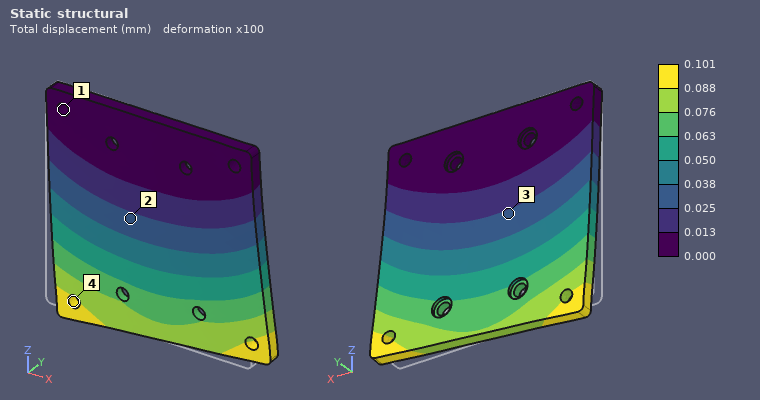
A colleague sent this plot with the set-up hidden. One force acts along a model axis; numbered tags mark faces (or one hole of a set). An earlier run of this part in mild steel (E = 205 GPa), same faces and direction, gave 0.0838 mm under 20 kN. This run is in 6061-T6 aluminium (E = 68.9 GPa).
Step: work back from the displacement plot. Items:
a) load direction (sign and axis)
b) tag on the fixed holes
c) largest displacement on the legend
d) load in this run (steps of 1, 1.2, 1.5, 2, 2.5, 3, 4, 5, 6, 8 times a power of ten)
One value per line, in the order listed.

+X
1
0.101 mm
8 kN
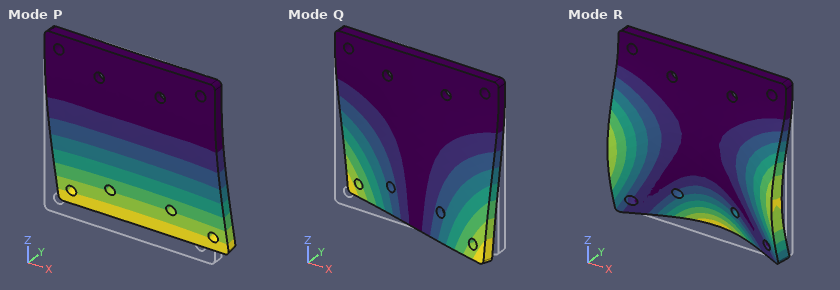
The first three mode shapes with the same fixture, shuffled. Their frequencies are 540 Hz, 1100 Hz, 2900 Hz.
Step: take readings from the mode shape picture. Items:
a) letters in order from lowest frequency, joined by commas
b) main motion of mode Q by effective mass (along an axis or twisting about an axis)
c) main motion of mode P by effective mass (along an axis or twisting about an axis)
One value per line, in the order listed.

P, Q, R
twisting about Z
along Y
